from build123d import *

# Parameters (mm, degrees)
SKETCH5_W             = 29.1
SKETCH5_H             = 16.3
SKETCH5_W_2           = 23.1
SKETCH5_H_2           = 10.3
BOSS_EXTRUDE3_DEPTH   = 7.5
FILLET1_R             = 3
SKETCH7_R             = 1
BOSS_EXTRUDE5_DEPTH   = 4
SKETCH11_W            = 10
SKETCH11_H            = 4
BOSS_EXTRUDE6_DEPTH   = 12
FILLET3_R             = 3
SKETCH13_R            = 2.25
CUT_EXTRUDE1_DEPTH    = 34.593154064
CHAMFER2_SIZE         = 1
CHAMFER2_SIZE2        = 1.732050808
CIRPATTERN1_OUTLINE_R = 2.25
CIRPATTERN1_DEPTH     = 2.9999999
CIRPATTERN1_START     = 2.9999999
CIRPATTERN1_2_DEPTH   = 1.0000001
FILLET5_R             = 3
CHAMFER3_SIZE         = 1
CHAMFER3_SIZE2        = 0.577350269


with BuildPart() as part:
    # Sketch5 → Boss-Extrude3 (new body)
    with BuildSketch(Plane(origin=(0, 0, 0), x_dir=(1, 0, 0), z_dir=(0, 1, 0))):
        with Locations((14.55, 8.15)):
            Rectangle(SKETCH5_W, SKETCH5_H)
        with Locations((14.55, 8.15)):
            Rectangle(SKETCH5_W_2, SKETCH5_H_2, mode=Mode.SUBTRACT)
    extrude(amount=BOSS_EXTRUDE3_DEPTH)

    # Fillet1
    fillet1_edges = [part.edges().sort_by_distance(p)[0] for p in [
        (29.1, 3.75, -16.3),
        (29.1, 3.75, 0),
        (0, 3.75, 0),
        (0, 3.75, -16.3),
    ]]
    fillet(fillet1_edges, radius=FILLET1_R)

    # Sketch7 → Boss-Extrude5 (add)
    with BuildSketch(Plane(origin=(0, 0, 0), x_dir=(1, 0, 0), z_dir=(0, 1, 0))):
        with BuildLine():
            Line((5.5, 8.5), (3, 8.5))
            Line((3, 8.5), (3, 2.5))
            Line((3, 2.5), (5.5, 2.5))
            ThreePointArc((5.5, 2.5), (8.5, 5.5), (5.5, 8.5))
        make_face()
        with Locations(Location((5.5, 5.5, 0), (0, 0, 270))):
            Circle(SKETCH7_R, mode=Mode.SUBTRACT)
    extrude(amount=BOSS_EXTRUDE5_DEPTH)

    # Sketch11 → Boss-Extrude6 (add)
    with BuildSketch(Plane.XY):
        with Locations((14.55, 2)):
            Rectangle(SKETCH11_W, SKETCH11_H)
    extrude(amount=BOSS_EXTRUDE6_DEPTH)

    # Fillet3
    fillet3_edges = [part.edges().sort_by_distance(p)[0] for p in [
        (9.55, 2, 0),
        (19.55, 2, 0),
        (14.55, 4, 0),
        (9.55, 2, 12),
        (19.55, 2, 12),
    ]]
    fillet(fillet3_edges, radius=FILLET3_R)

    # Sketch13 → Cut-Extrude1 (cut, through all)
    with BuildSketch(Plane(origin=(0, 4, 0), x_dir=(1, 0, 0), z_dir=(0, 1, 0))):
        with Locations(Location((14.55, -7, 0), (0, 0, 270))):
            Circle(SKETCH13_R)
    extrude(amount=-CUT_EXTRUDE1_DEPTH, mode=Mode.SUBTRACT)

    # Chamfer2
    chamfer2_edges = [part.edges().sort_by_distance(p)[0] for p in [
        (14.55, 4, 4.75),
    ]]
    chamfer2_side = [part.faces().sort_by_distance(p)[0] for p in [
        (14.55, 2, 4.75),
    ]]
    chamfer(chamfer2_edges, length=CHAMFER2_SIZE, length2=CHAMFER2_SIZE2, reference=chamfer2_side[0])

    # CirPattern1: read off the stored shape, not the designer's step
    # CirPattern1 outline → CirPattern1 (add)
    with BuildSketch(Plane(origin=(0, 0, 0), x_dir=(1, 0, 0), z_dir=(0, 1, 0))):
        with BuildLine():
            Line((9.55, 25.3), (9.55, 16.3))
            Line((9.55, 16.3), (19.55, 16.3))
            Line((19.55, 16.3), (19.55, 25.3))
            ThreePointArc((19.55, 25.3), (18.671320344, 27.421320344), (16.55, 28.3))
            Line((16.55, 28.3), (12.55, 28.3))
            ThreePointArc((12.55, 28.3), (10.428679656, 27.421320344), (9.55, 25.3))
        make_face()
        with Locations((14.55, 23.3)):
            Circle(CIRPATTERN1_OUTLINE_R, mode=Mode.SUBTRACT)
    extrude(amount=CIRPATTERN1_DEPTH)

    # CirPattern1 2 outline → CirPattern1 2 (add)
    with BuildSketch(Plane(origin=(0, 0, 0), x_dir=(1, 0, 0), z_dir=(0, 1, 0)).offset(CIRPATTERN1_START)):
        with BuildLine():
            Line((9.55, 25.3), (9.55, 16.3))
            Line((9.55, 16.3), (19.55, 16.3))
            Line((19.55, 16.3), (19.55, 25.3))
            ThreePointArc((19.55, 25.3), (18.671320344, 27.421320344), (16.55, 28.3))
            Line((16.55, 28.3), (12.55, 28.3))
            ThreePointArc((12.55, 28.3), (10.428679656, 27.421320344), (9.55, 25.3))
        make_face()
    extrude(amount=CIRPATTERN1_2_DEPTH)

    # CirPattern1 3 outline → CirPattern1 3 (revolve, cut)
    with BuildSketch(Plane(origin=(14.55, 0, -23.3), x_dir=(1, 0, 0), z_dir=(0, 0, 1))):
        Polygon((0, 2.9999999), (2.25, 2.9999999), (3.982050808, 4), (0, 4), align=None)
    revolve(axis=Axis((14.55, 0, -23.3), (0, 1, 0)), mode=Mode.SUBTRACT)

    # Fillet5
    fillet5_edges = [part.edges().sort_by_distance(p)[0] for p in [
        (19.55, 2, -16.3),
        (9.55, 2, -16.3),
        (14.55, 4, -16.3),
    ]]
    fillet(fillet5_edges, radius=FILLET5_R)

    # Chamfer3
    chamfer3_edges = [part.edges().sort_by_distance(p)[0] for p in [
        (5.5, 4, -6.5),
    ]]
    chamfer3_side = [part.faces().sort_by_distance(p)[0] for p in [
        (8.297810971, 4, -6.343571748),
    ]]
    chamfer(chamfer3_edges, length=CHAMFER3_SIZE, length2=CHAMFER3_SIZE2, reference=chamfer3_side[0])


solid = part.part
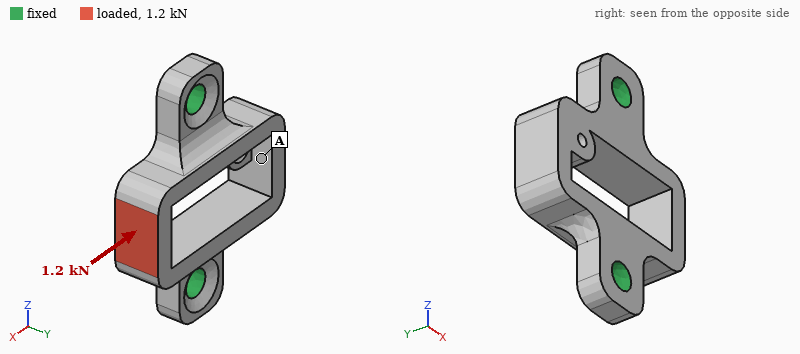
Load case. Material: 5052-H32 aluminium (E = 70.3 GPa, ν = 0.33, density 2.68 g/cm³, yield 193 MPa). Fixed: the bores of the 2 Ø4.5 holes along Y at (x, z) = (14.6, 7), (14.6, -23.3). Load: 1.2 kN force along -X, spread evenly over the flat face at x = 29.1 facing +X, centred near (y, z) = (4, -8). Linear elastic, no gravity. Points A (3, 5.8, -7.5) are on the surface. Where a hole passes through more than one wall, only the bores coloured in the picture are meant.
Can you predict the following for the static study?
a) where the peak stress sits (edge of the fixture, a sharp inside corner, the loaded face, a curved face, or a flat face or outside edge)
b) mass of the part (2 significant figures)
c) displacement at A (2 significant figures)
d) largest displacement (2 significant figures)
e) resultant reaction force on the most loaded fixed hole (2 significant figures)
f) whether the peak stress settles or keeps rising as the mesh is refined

edge of the fixture
7.1 g
18 µm
44 µm
640 N
keeps rising
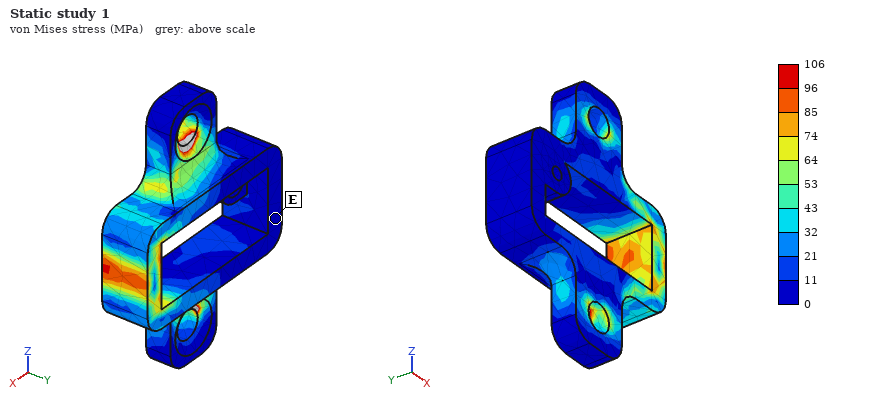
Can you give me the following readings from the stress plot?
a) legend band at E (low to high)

0 to 11 MPa
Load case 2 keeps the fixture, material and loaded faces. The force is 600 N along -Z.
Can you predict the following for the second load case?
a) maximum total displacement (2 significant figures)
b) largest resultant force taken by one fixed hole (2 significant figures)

28 µm
400 N
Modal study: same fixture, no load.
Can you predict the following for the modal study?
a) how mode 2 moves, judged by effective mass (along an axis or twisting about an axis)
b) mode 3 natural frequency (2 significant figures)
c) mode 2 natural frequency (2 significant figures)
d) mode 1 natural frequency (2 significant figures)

along Y
20 kHz
14 kHz
8700 Hz
